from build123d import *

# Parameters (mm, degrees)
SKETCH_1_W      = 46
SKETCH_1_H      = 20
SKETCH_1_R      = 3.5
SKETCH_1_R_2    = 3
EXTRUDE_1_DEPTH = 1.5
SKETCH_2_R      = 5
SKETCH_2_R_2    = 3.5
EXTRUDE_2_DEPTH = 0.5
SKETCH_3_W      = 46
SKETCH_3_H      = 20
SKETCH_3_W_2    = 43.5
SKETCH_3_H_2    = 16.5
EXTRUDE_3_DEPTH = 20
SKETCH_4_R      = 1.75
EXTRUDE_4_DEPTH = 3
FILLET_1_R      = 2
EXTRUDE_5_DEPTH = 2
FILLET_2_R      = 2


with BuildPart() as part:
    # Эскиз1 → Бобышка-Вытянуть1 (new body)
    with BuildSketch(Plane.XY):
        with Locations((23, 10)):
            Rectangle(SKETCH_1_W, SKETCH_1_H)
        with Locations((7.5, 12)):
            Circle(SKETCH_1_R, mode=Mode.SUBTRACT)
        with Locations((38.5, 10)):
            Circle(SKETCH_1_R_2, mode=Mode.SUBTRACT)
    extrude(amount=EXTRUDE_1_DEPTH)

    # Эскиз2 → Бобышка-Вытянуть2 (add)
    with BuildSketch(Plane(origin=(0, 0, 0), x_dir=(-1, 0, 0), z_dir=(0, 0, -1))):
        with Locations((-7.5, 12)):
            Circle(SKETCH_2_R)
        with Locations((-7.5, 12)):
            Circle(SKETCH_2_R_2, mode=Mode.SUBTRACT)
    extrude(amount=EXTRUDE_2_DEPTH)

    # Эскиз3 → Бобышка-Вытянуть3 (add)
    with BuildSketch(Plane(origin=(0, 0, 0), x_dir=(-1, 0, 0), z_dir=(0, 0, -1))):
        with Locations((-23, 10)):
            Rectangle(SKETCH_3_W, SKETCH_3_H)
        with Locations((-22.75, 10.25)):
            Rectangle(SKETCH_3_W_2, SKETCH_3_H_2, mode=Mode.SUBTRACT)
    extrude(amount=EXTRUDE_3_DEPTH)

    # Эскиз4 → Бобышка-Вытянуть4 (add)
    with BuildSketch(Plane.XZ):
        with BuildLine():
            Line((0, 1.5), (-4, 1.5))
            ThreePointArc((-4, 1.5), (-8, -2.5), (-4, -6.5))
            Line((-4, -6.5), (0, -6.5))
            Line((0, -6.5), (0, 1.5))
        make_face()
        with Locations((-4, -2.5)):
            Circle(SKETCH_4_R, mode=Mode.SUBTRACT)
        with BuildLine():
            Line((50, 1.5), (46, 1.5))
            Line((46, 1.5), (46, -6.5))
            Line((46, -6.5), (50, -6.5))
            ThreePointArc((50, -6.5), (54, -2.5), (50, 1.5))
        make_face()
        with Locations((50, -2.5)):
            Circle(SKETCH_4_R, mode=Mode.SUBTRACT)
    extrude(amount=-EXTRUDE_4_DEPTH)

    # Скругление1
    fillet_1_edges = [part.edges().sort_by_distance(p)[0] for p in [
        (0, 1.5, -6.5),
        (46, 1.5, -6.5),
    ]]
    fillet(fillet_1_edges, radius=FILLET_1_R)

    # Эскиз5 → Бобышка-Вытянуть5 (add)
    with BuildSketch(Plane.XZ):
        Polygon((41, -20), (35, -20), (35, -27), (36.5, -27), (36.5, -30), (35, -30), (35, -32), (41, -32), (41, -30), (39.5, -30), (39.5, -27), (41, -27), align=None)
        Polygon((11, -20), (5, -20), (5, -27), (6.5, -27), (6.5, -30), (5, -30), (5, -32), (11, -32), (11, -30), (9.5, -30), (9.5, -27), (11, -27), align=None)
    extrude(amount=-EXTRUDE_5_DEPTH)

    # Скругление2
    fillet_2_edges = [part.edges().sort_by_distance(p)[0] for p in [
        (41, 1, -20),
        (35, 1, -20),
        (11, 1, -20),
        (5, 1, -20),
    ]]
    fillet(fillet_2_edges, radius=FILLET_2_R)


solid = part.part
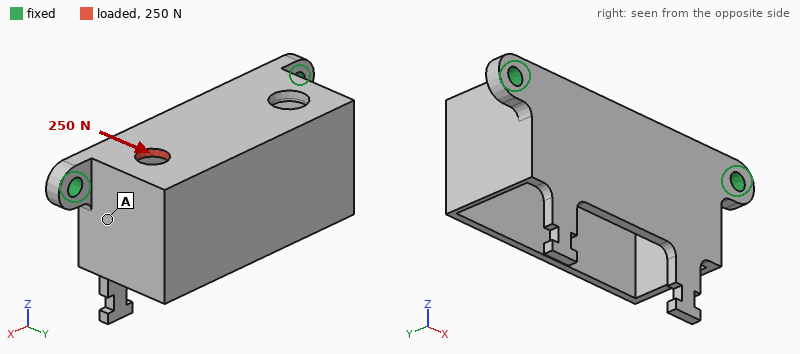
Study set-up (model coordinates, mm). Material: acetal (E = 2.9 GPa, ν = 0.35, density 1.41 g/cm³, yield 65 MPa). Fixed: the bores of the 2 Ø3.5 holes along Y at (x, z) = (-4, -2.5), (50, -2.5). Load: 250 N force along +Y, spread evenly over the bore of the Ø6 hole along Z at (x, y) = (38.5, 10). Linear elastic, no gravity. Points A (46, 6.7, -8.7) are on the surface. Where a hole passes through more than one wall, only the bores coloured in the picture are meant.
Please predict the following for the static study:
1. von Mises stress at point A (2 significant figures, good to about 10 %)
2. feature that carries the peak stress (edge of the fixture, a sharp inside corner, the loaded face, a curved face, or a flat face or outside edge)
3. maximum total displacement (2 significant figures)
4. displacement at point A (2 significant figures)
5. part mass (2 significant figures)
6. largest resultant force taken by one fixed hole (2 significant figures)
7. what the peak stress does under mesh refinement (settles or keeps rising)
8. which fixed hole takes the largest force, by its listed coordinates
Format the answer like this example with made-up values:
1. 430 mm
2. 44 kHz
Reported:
1. 4.7 MPa
2. edge of the fixture
3. 0.74 mm
4. 0.17 mm
5. 8.3 g
6. 210 N
7. keeps rising
8. (50, -2.5)
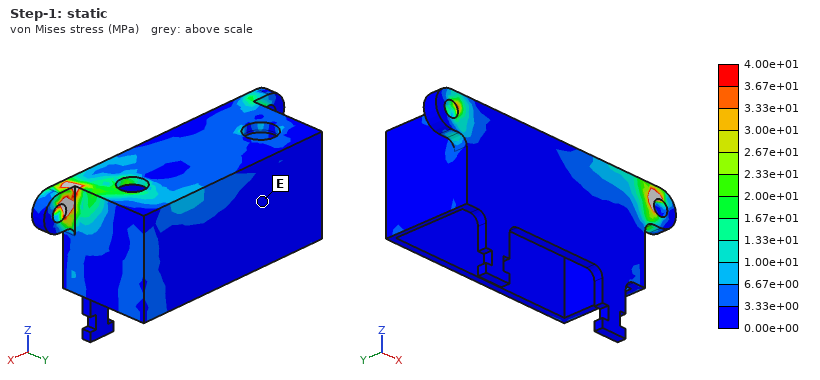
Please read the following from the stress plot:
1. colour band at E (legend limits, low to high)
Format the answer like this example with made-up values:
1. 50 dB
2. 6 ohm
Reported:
1. 0.00e+00 to 3.33e+00 MPa
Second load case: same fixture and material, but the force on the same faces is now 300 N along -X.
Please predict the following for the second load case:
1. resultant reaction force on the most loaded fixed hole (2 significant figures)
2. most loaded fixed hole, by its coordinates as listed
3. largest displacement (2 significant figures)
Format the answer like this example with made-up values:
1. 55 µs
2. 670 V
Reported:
1. 190 N
2. (50, -2.5)
3. 0.20 mm
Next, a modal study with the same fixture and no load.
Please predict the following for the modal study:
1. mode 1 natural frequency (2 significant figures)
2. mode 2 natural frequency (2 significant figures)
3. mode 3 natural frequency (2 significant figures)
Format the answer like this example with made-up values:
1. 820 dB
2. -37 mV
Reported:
1. 700 Hz
2. 1100 Hz
3. 1200 Hz
